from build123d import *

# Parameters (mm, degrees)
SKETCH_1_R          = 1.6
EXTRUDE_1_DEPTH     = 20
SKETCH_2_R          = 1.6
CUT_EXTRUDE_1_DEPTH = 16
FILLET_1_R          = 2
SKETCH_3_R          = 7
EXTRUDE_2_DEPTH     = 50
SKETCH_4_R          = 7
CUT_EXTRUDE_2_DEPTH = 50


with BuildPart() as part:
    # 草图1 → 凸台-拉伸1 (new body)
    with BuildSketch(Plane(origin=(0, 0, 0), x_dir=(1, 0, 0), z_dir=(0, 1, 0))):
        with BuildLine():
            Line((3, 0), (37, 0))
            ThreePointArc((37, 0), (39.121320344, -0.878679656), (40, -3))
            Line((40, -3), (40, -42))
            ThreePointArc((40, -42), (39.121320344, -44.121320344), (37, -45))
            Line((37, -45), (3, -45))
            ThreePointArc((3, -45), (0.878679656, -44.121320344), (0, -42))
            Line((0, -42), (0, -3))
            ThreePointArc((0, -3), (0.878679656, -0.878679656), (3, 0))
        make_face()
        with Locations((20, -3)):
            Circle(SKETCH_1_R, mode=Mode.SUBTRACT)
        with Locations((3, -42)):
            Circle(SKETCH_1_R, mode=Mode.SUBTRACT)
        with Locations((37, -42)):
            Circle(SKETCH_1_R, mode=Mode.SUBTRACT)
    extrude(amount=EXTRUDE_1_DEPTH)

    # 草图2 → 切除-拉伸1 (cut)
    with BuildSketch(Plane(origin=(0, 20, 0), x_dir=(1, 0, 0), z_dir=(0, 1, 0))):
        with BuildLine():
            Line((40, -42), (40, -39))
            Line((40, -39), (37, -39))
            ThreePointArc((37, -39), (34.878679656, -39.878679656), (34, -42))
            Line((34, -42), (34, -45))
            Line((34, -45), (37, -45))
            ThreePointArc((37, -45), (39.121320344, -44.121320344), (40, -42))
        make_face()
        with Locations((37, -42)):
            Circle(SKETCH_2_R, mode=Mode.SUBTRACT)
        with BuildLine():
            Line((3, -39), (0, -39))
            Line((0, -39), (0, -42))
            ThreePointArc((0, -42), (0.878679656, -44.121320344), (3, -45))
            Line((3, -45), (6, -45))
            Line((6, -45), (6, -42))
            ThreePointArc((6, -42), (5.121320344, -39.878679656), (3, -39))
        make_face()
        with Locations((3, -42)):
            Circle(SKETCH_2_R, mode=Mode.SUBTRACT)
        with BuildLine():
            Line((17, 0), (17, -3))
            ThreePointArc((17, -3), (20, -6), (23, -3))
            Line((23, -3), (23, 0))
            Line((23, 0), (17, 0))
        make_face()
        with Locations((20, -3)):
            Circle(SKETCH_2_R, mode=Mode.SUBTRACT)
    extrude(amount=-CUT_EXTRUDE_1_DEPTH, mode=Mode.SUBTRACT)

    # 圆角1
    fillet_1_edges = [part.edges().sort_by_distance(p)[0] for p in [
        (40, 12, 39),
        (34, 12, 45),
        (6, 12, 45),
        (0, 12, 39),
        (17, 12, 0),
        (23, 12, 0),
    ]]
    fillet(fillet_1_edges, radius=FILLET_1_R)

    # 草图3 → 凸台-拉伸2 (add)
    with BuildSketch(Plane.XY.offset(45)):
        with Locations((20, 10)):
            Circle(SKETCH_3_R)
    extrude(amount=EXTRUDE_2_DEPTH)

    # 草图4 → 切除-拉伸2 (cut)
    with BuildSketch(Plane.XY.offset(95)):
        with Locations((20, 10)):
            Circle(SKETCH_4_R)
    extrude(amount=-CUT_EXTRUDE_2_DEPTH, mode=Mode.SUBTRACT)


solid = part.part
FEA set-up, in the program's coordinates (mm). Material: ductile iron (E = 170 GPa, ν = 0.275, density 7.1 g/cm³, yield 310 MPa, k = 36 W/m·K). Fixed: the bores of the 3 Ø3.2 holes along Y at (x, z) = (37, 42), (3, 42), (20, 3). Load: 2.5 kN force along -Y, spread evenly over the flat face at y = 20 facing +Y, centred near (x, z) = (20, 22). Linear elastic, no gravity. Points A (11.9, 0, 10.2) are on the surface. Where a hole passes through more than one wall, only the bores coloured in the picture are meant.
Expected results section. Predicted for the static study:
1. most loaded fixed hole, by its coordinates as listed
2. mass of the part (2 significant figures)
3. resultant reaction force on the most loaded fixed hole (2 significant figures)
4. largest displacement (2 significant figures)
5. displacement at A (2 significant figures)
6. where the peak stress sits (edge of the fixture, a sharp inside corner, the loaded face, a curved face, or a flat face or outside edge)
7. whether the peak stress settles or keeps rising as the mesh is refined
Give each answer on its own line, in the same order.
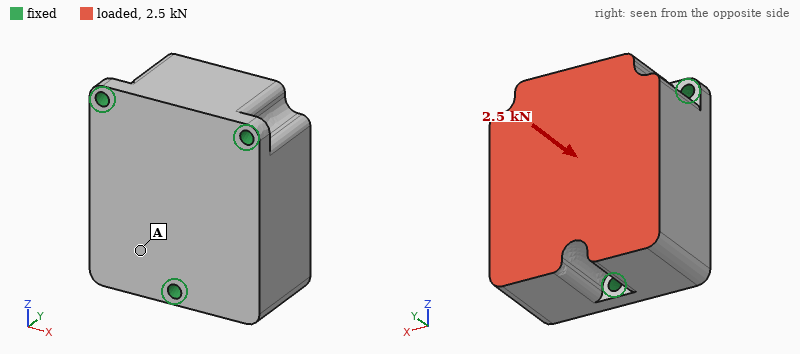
(20, 3)
240 g
1.3 kN
2.3 µm
1.9 µm
edge of the fixture
keeps rising
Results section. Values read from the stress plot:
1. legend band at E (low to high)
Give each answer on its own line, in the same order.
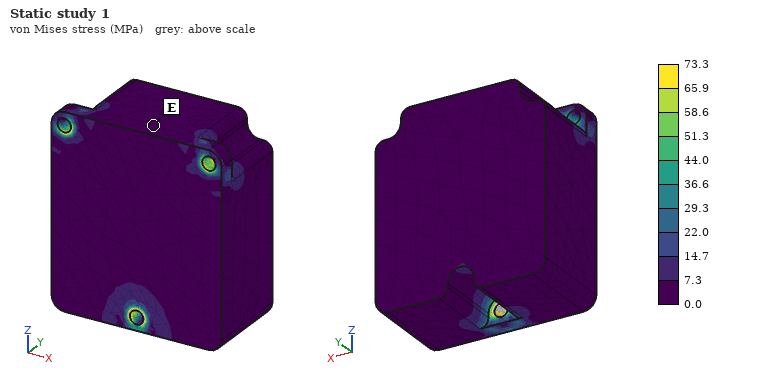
0.0 to 7.3 MPa
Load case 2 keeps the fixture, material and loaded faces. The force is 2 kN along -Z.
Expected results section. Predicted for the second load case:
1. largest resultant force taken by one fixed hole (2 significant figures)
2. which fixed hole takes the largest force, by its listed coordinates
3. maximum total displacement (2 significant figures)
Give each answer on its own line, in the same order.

1.3 kN
(20, 3)
2.8 µm
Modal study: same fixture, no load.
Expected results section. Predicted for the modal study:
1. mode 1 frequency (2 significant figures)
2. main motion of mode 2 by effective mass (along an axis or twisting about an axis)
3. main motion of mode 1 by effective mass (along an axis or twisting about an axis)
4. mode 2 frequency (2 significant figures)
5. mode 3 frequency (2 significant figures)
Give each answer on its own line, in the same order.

9000 Hz
along Y
along X
12 kHz
14 kHz
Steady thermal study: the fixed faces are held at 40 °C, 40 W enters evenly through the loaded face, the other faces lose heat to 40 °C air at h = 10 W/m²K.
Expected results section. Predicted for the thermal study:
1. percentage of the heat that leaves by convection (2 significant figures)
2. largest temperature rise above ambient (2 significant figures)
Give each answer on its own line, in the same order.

4.7 %
48 K
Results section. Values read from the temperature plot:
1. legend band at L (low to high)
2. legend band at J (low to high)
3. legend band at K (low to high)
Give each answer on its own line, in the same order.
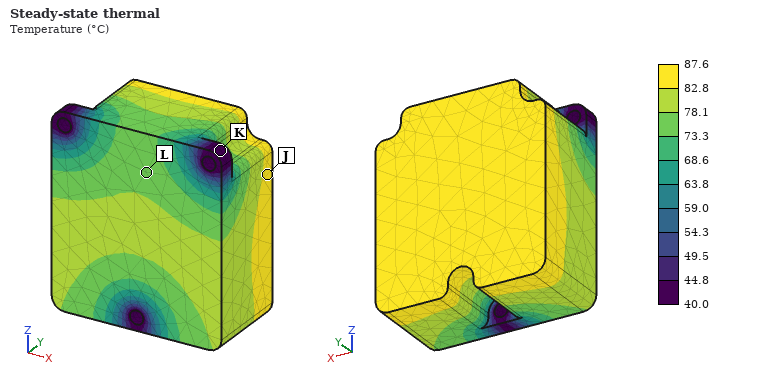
73.3 to 78.1 °C
82.8 to 87.6 °C
40.0 to 44.8 °C
